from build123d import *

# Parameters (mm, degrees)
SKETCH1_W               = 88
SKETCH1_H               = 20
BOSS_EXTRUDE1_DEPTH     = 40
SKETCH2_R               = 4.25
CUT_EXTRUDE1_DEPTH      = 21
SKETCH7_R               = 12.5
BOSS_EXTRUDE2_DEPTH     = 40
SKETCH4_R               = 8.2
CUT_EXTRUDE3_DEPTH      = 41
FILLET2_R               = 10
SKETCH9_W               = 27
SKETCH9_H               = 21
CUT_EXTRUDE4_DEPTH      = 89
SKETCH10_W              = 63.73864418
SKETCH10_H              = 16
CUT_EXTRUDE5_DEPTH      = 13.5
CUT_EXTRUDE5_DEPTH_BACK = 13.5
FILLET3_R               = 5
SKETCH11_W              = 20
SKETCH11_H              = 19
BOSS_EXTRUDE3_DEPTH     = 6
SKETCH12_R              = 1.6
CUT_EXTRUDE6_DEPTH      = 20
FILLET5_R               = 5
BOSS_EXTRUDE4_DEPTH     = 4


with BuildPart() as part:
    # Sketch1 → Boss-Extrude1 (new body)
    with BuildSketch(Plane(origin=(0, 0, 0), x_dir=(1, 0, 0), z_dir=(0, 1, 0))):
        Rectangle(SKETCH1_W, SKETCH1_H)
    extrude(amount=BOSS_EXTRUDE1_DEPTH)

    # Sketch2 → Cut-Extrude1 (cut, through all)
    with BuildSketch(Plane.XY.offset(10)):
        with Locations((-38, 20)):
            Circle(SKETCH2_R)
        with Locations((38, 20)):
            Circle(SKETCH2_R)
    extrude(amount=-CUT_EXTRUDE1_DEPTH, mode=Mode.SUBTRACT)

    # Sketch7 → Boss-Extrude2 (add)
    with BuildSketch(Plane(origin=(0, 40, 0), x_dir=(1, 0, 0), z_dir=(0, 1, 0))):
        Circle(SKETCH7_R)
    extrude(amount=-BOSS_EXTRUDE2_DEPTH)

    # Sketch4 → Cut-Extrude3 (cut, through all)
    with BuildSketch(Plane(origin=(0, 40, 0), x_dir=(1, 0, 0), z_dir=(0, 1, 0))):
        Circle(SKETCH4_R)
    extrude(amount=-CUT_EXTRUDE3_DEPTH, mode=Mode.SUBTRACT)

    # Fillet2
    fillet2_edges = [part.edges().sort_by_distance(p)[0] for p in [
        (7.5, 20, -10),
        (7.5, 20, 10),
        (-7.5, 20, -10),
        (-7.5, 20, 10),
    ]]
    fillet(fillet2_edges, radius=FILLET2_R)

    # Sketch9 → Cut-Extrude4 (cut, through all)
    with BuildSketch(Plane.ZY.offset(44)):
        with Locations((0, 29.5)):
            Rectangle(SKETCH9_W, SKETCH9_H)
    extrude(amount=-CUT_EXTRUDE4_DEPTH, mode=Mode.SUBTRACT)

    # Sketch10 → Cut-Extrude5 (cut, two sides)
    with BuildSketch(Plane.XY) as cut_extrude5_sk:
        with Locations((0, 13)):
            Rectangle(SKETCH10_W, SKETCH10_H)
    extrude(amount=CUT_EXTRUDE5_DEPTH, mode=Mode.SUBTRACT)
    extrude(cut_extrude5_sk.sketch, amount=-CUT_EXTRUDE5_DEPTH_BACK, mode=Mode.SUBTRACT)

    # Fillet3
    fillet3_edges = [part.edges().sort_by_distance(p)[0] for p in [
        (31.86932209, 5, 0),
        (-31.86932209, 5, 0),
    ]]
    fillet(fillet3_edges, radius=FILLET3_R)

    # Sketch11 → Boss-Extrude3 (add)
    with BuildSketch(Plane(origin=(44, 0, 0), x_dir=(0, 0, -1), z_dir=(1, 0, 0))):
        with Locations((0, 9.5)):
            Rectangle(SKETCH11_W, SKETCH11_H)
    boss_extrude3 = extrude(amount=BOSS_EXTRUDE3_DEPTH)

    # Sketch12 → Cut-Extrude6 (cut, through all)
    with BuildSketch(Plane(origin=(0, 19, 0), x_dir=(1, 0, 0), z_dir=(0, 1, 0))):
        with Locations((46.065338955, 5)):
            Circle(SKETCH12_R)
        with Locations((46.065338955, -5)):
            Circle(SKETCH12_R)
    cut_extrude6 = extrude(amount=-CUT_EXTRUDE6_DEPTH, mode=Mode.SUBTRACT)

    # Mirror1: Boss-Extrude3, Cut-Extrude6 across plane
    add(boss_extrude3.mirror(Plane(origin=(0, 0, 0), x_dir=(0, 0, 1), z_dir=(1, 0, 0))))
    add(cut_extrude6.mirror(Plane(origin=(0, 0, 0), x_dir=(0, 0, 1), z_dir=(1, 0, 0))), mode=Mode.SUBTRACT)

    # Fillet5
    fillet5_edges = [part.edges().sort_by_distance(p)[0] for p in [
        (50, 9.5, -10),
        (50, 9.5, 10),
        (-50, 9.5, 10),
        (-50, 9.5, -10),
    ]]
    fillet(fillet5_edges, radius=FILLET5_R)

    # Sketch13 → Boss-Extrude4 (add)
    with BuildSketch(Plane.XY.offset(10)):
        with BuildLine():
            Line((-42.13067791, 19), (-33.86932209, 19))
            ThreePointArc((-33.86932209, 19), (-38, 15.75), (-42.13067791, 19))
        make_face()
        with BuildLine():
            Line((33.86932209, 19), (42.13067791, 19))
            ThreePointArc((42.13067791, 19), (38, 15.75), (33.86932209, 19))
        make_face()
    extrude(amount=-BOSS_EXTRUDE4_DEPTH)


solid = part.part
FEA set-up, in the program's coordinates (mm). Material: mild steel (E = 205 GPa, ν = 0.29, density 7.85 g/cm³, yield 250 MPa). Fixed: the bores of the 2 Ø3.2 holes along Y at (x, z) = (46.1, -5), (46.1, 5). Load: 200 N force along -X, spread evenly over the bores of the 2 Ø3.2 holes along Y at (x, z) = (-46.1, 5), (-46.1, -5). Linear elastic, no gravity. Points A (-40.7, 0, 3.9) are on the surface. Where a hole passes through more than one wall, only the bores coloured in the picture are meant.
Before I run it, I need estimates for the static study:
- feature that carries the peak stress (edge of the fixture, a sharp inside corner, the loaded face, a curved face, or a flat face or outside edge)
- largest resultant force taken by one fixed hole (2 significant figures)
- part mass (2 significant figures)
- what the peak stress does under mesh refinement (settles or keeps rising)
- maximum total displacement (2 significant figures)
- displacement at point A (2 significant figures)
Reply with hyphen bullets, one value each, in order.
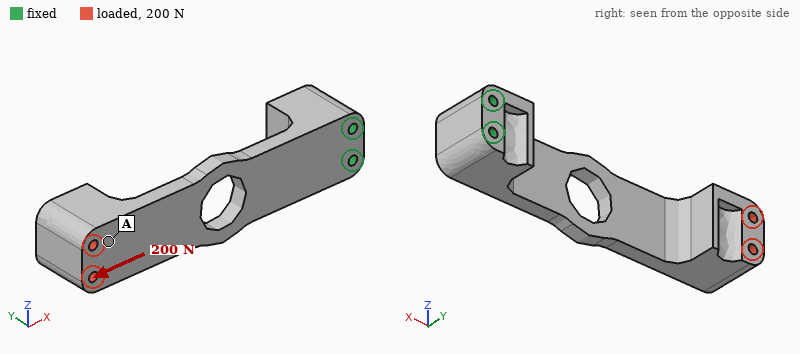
- a sharp inside corner
- 100 N
- 140 g
- keeps rising
- 0.16 mm
- 0.12 mm
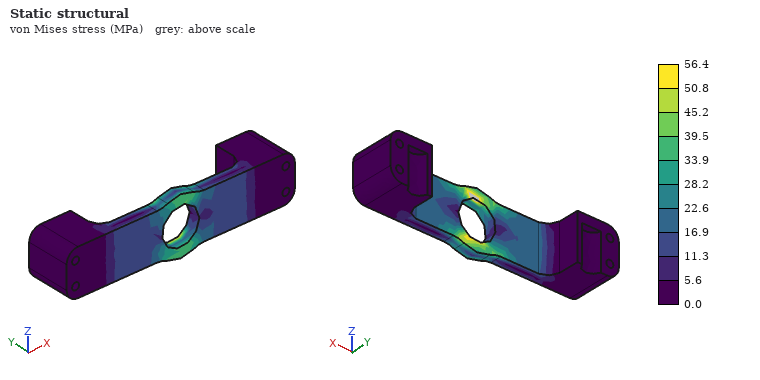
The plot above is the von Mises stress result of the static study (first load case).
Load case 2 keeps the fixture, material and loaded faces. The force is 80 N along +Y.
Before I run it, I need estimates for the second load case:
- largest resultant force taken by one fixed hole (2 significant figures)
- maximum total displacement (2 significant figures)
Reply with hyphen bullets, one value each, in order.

- 43 N
- 0.46 mm
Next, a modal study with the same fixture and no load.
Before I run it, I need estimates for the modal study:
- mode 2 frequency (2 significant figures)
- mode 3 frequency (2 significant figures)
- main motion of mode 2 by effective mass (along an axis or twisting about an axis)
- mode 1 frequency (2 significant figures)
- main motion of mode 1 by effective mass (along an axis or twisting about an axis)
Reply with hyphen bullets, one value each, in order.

- 1100 Hz
- 2400 Hz
- along Z
- 330 Hz
- along Y
